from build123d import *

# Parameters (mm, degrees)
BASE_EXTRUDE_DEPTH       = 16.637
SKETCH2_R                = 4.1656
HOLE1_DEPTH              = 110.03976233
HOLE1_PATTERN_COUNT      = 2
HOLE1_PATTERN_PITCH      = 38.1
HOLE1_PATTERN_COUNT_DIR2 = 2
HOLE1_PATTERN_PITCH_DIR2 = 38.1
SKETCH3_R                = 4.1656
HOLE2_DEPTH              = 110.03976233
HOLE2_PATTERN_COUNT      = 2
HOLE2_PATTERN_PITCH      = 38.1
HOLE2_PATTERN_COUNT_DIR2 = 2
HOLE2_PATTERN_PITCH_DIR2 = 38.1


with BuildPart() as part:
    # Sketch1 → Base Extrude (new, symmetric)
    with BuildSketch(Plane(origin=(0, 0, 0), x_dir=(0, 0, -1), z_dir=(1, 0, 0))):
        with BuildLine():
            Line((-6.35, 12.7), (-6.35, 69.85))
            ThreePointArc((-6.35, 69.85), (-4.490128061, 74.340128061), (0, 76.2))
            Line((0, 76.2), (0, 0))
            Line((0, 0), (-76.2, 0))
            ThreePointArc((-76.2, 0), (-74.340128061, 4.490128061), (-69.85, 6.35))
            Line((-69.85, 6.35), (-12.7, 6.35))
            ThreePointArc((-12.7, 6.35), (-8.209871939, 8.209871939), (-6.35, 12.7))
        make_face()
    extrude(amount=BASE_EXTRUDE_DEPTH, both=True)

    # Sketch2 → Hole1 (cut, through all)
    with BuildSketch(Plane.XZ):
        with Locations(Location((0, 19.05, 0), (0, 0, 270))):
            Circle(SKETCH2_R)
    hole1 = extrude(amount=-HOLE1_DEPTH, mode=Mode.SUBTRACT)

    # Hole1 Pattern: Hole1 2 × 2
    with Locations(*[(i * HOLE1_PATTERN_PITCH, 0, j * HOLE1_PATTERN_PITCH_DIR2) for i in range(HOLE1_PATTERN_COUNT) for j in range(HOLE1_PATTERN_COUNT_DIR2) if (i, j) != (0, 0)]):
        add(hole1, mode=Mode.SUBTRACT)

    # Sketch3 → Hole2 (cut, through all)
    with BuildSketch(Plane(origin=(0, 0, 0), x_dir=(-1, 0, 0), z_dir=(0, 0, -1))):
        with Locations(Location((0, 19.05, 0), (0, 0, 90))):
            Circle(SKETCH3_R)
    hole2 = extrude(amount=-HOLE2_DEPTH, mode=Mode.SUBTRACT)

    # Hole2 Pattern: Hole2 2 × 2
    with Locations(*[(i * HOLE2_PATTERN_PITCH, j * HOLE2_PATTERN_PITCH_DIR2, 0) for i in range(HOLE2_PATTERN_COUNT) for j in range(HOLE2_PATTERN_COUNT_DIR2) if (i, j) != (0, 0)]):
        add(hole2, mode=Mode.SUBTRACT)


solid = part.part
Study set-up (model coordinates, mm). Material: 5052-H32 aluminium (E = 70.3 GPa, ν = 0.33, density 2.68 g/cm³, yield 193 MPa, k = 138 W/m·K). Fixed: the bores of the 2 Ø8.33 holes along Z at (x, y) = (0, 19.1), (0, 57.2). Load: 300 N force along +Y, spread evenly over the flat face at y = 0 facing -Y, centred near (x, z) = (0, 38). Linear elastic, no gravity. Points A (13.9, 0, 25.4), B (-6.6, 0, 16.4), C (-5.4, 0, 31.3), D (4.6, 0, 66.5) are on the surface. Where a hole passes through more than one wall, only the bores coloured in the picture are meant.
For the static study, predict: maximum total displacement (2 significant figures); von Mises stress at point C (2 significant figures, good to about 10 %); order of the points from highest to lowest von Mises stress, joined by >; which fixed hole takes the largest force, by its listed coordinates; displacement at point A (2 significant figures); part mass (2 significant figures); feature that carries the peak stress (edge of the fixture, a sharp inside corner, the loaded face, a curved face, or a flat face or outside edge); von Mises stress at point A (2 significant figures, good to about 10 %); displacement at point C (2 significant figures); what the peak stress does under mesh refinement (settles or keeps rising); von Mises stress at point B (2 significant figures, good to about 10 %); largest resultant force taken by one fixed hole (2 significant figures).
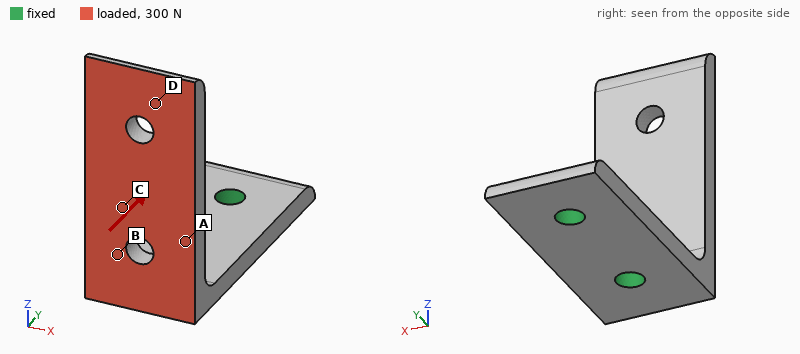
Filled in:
0.41 mm
17 MPa
B > A > C > D
(0, 19.1)
0.084 mm
78 g
edge of the fixture
26 MPa
0.12 mm
keeps rising
40 MPa
290 N
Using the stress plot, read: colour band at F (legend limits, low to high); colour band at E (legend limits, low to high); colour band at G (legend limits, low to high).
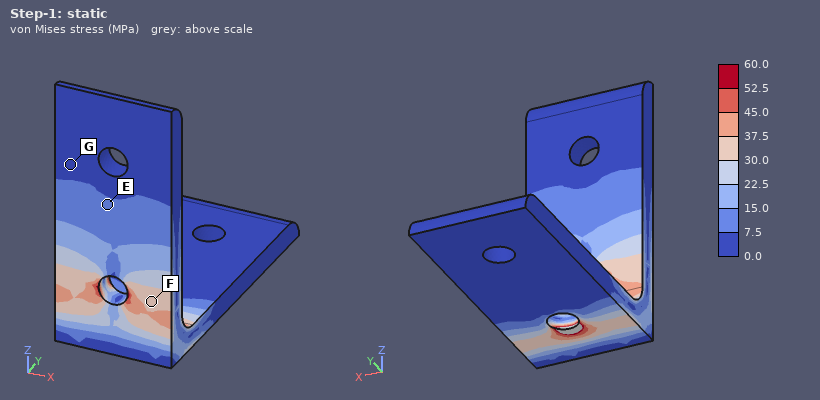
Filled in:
30.0 to 37.5 MPa
7.5 to 15.0 MPa
0.0 to 7.5 MPa
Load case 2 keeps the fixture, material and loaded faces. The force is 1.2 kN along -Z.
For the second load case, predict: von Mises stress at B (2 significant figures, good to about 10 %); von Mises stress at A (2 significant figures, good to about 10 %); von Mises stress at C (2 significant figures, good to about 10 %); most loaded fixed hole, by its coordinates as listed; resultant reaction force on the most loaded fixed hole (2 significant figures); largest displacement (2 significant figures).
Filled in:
23 MPa
17 MPa
13 MPa
(0, 19.1)
1.3 kN
0.36 mm
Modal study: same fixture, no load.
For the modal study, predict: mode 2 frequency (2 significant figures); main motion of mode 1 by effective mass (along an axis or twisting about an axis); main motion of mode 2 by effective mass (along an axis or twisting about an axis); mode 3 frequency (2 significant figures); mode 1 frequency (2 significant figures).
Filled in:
1600 Hz
along Y
along X
4200 Hz
860 Hz
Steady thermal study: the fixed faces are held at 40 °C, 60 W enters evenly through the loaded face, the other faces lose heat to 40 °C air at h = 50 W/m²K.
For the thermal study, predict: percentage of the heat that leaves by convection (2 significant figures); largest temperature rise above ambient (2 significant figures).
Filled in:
20 %
79 K
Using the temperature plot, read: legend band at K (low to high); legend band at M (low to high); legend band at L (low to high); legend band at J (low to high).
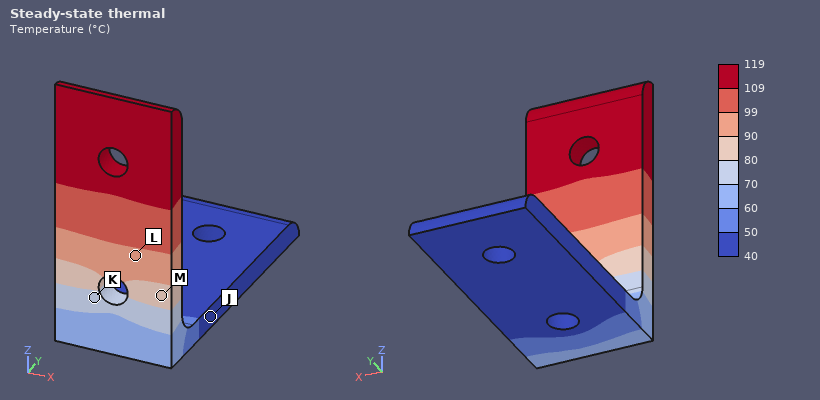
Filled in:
70 to 80 °C
80 to 90 °C
90 to 99 °C
40 to 50 °C
